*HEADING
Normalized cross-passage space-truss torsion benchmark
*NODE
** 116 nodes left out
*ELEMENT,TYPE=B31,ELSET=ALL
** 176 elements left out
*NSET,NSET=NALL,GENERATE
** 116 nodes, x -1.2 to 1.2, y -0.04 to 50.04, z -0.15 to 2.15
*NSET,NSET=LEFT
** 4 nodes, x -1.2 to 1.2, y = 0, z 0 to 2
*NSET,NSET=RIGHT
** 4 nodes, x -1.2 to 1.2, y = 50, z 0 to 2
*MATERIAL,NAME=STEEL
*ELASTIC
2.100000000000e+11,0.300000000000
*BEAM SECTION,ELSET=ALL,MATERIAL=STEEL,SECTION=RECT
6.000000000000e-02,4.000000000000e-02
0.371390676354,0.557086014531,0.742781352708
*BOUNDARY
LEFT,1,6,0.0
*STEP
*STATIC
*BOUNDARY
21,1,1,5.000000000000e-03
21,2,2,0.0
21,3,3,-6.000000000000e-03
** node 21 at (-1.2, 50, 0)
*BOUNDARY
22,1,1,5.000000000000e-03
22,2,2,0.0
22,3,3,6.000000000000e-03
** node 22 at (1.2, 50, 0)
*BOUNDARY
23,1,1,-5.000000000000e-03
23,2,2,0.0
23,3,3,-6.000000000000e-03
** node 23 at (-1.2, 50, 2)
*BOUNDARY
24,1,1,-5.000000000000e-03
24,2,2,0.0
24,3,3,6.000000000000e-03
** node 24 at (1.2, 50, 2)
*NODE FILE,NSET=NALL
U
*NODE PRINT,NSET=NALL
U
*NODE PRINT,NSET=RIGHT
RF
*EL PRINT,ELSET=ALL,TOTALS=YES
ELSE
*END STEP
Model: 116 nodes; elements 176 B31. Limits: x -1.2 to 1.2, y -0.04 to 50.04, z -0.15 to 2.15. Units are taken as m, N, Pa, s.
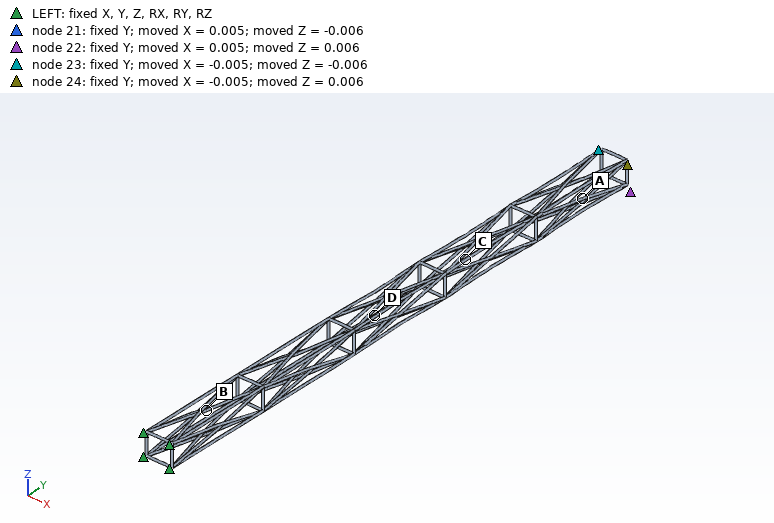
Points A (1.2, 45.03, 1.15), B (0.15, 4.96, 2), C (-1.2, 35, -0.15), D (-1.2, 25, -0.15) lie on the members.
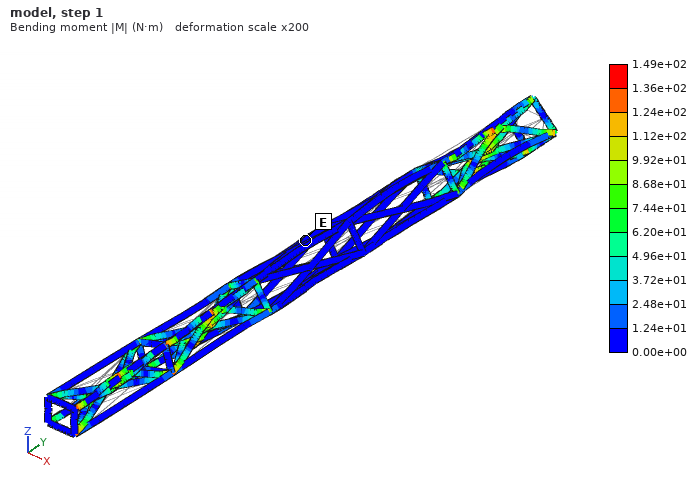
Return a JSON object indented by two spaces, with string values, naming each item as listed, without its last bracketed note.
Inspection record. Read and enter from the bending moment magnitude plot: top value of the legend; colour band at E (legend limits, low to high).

{
  "top value of the legend": "1.49e+02 N·m",
  "colour band at E": "0.00e+00 to 1.24e+01 N·m"
}
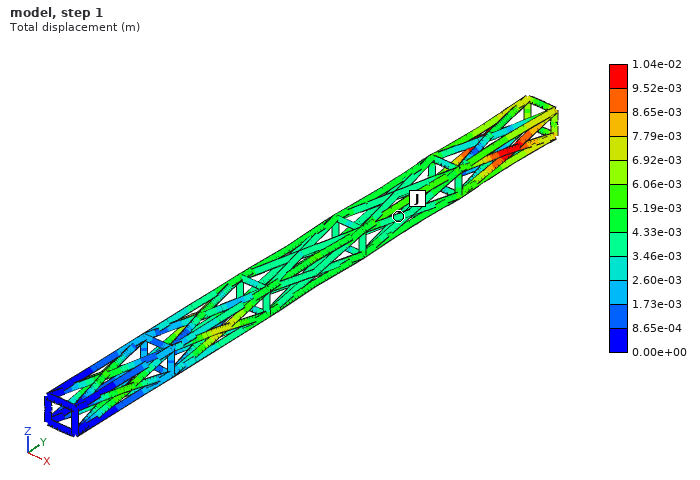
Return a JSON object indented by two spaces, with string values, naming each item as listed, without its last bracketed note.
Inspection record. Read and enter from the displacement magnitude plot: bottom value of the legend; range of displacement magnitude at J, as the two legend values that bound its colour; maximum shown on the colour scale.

{
  "bottom value of the legend": "0.00e+00 m",
  "range of displacement magnitude at J, as the two legend values that bound its colour": "3.46e-03 to 4.33e-03 m",
  "maximum shown on the colour scale": "1.04e-02 m"
}
